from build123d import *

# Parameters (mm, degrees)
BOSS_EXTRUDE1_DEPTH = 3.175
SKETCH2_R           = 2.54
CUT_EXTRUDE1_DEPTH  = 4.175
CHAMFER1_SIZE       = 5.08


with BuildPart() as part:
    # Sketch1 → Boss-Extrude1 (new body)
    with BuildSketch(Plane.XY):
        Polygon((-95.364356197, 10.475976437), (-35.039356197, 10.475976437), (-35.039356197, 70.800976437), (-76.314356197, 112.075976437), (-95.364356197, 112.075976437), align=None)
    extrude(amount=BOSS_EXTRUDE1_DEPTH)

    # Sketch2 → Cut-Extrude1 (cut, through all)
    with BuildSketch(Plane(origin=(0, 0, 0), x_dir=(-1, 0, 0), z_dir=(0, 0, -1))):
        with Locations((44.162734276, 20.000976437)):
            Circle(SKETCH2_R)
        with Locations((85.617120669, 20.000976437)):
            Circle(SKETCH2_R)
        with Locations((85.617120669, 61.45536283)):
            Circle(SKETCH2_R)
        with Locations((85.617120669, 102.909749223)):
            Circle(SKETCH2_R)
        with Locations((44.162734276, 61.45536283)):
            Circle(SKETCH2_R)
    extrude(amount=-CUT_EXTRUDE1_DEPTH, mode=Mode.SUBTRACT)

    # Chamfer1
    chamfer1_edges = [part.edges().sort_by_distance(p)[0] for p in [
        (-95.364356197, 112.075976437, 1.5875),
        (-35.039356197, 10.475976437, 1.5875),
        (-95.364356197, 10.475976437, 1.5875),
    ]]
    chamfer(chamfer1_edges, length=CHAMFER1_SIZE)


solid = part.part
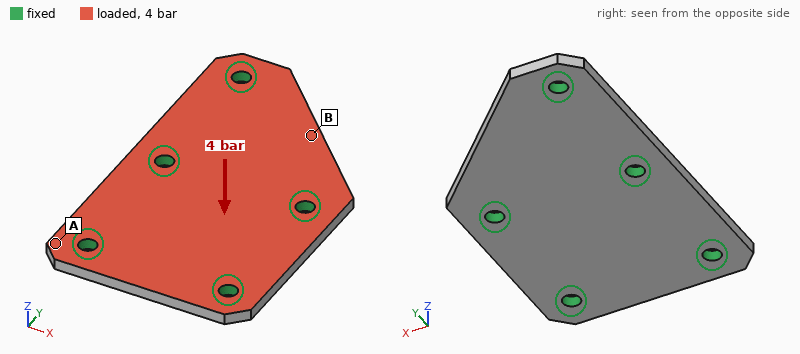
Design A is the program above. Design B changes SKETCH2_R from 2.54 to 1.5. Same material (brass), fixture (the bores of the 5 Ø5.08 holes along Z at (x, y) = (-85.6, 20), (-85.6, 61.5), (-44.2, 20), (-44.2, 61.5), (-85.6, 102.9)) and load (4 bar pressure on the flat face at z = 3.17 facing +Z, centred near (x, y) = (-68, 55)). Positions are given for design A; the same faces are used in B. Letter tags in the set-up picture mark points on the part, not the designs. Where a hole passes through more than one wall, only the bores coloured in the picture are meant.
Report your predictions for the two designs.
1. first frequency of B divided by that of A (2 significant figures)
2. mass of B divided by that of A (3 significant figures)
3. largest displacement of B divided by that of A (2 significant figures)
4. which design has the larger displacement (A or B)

0.89
1.01
1.2
B
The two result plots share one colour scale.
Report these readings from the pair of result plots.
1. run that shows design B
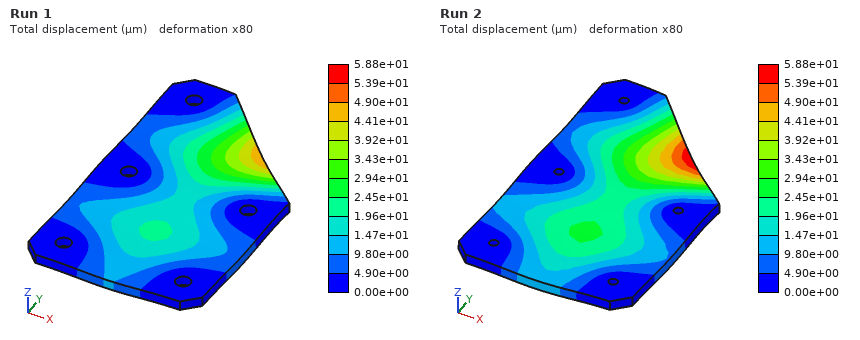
Run 2
